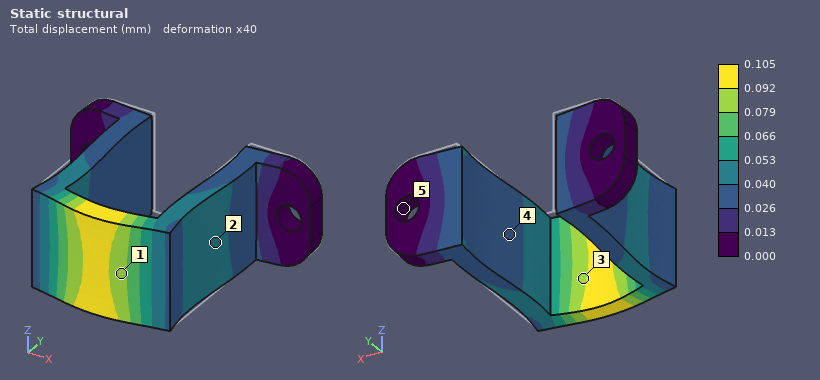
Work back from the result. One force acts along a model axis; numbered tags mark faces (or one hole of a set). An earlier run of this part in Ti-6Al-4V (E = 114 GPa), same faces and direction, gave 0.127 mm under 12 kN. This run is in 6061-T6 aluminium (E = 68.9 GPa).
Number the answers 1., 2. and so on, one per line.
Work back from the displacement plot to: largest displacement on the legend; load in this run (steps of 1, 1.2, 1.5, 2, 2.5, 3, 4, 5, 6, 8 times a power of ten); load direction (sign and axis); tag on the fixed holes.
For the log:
1. 0.105 mm
2. 6 kN
3. -Y
4. 5
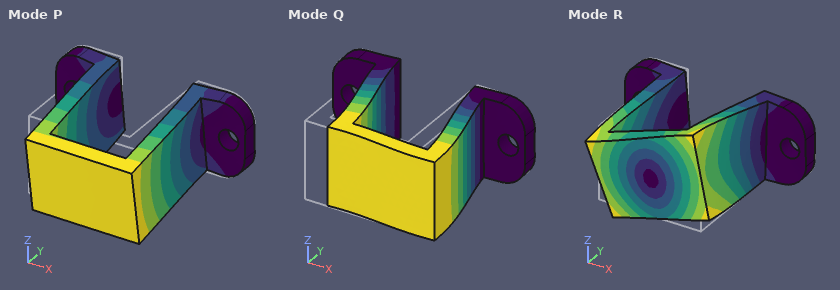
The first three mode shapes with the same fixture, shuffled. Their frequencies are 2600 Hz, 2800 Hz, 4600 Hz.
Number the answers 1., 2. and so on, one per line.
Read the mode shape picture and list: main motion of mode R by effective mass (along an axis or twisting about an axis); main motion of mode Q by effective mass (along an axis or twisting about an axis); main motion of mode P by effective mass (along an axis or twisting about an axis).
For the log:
1. twisting about Y
2. along X
3. along Z
